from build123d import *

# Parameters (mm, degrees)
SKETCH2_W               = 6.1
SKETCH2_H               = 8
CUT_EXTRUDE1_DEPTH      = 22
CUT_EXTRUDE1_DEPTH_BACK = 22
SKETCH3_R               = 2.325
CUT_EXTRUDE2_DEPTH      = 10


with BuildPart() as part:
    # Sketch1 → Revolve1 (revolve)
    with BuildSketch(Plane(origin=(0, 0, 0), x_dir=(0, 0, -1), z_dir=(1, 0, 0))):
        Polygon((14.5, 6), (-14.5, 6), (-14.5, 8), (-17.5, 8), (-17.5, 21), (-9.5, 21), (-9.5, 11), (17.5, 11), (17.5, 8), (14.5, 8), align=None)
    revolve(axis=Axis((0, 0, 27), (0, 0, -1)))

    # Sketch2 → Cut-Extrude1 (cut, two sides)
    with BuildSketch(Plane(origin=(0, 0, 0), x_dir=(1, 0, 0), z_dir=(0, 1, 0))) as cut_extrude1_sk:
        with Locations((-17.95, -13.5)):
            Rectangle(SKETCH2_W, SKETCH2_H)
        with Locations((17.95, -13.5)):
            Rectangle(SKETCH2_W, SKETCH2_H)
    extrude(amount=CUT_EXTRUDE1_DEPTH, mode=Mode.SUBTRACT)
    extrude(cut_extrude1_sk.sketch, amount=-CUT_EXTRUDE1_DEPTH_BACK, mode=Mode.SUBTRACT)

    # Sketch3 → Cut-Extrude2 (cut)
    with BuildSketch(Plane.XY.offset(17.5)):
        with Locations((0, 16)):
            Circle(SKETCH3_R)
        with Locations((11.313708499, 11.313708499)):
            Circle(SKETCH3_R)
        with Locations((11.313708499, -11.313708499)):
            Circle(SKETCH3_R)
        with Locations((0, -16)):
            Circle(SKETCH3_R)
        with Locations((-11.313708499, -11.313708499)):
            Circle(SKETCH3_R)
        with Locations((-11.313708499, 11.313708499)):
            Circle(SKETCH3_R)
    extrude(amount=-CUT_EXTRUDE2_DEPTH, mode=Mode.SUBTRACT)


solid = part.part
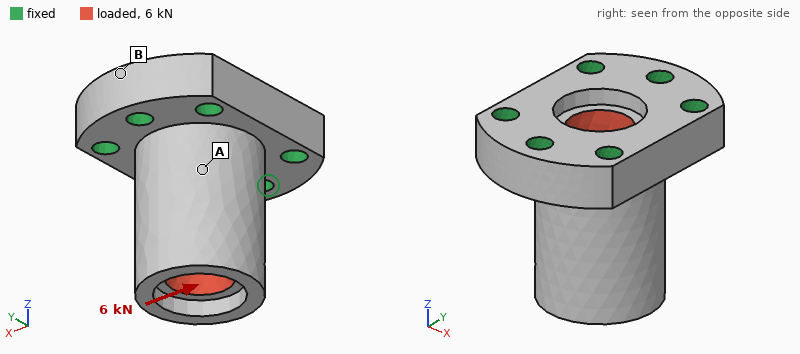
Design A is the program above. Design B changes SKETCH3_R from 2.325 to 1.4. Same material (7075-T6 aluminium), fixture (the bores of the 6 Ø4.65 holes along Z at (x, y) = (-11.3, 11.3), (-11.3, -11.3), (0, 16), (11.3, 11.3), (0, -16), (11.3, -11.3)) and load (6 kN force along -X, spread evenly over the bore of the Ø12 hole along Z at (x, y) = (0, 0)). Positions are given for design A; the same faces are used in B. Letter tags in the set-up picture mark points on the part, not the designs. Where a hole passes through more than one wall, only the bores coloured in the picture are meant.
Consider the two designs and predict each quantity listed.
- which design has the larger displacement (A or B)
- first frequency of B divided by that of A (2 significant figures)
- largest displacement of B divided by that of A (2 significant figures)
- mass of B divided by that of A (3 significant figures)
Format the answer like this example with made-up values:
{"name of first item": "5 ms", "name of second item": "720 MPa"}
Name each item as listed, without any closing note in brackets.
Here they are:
{"which design has the larger displacement": "B", "first frequency of B divided by that of A": "0.94", "largest displacement of B divided by that of A": "1.1", "mass of B divided by that of A": "1.04"}
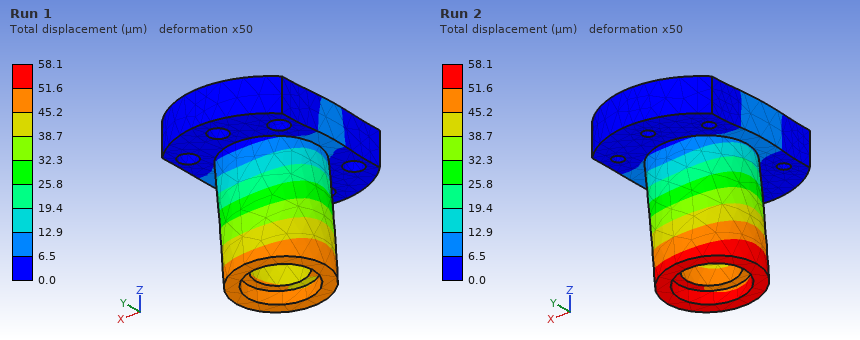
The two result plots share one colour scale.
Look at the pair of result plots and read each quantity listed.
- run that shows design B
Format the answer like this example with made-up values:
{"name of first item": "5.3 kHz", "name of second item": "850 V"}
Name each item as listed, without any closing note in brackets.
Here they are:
{"run that shows design B": "Run 2"}
